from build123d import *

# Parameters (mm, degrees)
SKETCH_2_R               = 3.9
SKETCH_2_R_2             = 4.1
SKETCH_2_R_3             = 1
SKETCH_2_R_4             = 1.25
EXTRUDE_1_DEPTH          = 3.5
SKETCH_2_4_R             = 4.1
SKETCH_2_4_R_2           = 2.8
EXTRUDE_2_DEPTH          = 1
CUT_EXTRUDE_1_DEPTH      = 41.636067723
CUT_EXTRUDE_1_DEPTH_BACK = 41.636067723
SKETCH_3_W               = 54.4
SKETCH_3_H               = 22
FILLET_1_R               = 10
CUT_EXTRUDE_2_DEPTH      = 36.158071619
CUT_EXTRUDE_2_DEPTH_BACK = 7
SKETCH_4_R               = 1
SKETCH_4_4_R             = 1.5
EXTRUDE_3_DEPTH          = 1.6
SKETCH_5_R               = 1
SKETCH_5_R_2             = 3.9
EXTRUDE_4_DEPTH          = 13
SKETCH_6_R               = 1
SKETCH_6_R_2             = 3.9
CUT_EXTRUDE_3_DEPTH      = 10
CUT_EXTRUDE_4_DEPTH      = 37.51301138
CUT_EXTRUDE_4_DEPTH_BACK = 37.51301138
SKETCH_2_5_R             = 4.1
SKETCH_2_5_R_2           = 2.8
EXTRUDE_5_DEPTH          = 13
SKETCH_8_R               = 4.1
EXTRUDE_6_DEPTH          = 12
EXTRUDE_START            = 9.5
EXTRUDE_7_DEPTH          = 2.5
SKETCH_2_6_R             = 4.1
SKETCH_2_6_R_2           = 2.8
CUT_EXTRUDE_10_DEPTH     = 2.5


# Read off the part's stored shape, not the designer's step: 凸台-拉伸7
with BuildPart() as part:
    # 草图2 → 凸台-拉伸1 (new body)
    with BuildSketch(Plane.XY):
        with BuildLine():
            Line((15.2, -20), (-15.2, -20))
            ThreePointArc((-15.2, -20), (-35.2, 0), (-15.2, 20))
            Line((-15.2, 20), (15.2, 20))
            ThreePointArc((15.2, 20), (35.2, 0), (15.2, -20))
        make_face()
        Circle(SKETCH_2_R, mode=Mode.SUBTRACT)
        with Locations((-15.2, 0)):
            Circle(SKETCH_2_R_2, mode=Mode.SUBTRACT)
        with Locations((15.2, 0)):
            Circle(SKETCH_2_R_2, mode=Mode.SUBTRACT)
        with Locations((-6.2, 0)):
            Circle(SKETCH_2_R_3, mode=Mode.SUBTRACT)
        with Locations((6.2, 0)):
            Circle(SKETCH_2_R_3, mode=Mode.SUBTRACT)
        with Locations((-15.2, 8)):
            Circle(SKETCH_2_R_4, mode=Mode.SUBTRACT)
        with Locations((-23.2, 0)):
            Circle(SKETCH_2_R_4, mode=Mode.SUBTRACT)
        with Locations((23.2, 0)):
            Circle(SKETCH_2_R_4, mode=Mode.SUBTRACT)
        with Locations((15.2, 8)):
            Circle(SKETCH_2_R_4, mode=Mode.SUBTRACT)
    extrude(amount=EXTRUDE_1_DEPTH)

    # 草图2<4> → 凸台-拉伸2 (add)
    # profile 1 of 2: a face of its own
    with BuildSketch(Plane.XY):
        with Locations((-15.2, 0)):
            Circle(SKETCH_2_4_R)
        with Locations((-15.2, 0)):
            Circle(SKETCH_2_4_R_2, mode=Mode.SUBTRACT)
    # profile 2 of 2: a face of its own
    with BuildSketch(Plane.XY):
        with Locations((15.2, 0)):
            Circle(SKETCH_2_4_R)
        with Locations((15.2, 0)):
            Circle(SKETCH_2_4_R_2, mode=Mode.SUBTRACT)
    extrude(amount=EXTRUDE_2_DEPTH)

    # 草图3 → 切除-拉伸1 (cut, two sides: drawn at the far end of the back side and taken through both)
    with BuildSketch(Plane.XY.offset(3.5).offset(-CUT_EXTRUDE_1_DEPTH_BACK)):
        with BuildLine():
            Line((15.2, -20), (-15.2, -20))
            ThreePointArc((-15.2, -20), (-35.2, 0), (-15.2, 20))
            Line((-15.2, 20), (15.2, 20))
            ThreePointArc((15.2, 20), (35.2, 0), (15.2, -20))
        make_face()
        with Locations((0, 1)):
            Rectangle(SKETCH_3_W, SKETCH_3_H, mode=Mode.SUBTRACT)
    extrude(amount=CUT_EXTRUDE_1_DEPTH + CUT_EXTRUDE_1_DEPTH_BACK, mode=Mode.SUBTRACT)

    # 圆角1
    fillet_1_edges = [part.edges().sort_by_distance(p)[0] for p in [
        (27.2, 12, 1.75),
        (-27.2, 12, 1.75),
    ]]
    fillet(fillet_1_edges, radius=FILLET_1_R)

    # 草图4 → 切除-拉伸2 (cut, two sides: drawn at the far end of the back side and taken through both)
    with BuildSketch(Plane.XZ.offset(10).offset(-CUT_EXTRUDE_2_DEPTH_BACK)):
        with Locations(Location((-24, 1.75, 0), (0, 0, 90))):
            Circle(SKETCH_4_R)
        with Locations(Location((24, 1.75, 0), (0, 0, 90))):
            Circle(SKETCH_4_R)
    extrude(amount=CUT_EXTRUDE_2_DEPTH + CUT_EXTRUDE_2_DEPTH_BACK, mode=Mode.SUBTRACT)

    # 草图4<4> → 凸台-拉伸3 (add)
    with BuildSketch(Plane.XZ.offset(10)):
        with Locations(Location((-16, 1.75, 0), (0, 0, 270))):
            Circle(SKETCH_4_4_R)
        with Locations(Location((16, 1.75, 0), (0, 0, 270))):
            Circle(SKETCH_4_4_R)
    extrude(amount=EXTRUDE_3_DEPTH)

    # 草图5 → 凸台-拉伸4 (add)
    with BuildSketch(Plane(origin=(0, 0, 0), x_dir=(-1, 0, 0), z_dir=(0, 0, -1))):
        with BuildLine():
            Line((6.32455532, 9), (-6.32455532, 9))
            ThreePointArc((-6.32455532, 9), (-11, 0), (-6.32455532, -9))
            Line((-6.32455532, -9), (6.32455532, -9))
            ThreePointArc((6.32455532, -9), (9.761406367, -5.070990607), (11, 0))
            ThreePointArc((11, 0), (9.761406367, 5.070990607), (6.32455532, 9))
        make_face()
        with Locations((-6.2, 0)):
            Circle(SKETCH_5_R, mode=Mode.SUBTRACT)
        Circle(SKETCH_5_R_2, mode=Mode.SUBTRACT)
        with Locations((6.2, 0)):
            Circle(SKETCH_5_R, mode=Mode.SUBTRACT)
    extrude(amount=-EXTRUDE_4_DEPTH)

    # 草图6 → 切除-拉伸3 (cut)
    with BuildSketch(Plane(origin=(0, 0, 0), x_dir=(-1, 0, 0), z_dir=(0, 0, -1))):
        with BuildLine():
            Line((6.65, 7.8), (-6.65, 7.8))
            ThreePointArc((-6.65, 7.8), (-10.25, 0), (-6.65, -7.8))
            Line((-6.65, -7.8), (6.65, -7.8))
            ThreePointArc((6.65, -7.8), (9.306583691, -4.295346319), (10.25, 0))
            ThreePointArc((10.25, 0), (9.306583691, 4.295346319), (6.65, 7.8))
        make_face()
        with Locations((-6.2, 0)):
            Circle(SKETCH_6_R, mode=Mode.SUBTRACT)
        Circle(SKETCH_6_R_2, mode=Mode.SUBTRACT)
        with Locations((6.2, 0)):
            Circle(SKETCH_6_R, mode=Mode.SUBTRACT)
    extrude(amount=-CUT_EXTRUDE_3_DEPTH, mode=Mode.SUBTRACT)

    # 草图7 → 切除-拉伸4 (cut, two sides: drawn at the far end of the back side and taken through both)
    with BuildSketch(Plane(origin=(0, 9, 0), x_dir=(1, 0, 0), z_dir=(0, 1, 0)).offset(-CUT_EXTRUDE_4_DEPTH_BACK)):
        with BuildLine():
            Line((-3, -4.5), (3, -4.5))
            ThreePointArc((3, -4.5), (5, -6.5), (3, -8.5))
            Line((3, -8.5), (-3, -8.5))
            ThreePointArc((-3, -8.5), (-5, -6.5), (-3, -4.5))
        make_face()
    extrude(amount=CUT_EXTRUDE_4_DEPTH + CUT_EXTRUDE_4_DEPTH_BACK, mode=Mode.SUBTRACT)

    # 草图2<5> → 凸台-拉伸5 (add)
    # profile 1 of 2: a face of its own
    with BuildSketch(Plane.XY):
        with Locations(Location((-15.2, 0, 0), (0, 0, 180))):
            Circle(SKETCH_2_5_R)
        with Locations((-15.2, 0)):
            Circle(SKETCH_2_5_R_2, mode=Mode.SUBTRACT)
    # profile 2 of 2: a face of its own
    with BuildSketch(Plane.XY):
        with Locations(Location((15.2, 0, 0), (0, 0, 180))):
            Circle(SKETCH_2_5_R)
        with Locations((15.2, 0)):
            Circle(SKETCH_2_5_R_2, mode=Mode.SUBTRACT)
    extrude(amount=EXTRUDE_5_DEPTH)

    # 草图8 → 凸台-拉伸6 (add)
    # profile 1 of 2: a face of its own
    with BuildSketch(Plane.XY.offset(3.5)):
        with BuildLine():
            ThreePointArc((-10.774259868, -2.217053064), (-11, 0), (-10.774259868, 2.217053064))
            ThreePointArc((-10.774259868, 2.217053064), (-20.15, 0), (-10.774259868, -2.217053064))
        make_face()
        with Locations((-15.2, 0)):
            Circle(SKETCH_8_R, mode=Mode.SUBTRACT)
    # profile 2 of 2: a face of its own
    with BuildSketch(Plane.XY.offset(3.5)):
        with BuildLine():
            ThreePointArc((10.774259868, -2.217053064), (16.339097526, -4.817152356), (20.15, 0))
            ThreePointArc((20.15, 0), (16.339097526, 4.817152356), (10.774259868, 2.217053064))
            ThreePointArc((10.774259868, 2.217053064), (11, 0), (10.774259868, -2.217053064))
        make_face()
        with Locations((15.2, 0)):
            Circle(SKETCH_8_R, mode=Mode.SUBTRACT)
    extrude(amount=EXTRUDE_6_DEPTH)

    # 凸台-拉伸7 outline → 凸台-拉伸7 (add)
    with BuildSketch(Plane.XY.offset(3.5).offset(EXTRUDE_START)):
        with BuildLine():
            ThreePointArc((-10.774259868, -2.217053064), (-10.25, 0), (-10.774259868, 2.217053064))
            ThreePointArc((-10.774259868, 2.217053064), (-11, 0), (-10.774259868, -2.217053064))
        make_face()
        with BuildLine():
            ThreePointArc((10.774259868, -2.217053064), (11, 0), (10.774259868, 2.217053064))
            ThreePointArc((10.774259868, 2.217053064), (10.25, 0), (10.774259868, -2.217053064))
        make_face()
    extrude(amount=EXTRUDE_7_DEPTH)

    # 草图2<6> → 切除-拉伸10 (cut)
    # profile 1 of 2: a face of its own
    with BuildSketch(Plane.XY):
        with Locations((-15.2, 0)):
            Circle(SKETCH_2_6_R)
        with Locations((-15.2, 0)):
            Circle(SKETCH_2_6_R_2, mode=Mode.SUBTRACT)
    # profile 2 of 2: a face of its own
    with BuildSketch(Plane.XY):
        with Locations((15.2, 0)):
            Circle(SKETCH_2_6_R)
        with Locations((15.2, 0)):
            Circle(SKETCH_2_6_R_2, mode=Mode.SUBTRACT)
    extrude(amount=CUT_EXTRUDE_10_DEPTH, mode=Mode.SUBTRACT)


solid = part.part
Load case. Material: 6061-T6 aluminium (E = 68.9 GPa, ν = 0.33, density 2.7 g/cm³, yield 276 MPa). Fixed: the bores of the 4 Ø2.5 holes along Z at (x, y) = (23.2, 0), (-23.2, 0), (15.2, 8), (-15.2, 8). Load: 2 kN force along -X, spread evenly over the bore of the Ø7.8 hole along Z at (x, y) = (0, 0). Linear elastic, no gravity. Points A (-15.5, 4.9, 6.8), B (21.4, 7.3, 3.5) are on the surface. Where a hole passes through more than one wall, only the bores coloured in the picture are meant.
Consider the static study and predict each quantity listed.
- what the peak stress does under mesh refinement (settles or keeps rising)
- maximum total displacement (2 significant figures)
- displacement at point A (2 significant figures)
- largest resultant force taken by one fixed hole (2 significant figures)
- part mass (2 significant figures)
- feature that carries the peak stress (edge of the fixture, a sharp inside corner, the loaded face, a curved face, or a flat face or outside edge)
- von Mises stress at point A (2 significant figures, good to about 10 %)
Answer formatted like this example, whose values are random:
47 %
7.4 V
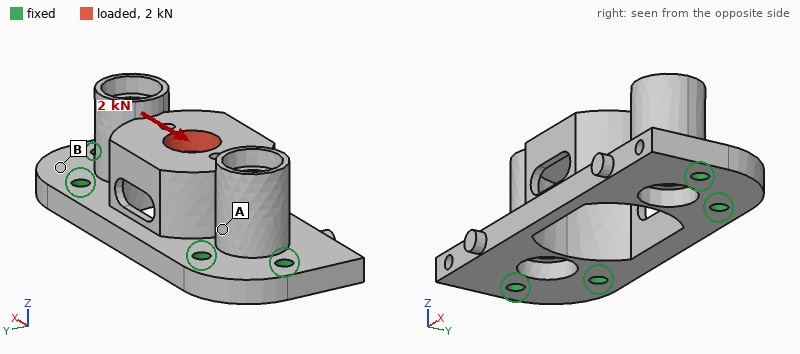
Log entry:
keeps rising
25 µm
8.0 µm
770 N
13 g
a sharp inside corner
28 MPa
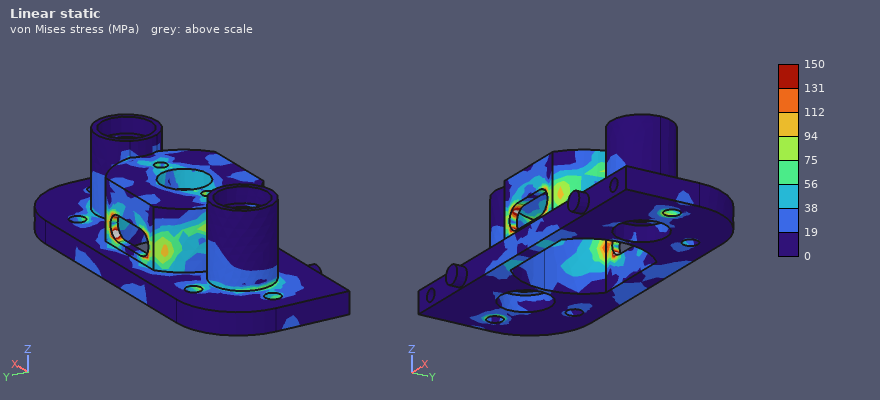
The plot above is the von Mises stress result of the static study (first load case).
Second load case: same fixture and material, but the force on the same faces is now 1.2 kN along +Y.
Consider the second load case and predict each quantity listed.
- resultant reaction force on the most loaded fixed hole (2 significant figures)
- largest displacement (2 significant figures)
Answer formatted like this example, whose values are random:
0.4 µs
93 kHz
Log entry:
740 N
73 µm
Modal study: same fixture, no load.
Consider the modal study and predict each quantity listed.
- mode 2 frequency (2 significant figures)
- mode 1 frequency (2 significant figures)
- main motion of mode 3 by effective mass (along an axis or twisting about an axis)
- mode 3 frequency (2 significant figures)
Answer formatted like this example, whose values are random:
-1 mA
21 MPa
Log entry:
19 kHz
9400 Hz
along Z
21 kHz
